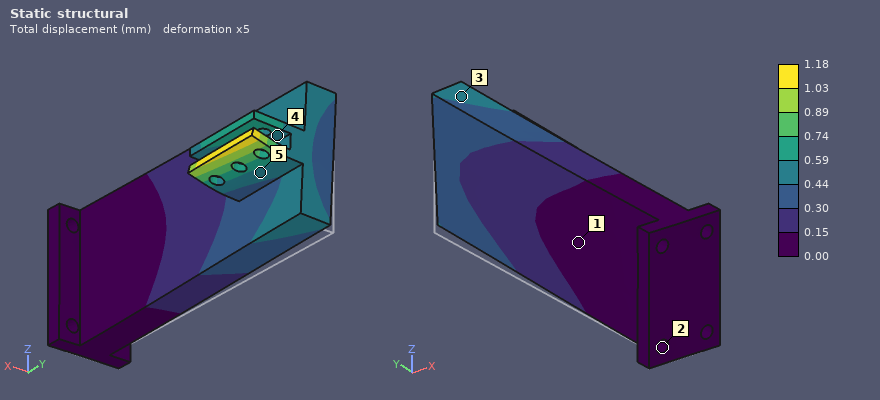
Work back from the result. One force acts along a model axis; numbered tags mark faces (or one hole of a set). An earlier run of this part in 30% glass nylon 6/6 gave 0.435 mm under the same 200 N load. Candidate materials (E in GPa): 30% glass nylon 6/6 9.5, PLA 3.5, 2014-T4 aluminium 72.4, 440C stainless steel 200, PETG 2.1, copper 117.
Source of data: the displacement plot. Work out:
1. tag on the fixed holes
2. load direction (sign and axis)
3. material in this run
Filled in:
2
+Z
PLA
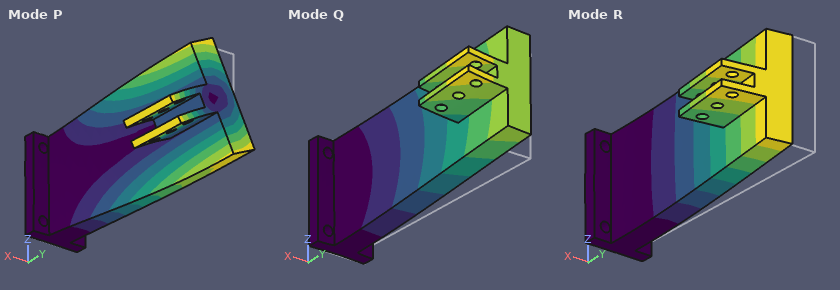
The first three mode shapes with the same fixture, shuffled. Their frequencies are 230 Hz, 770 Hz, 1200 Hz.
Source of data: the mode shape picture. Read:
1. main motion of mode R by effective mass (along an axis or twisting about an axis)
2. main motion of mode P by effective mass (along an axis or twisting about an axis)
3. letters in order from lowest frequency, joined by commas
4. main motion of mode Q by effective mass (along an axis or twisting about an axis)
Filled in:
along X
twisting about Y
R, Q, P
along Z
